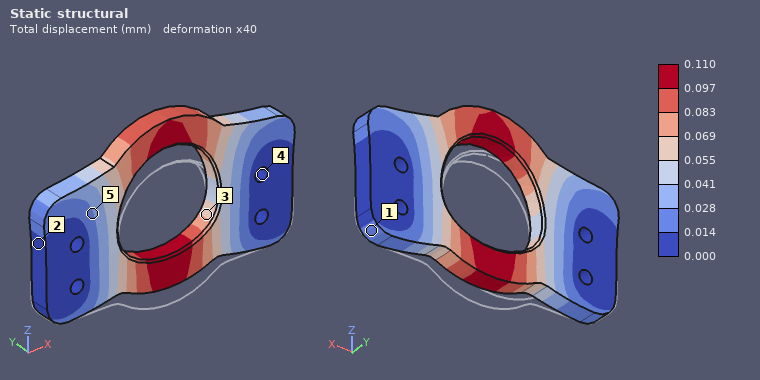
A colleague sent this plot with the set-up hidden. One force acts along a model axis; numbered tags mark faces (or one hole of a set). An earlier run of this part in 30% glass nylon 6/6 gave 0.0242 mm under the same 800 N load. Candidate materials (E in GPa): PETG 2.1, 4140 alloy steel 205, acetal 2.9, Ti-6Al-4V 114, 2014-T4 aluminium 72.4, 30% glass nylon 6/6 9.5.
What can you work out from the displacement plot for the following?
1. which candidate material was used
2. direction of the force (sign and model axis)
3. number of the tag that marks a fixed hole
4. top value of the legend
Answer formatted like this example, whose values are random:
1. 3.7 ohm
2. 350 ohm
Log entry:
1. PETG
2. +Z
3. 4
4. 0.110 mm
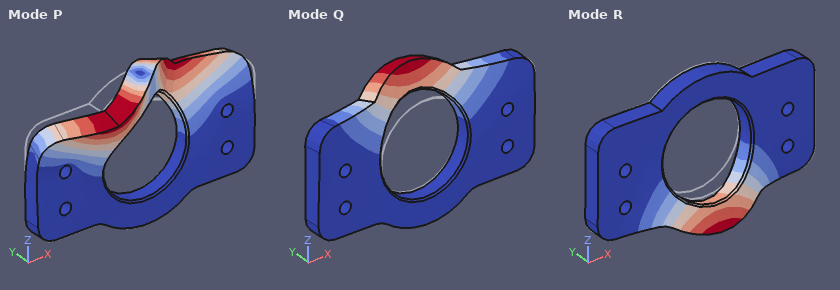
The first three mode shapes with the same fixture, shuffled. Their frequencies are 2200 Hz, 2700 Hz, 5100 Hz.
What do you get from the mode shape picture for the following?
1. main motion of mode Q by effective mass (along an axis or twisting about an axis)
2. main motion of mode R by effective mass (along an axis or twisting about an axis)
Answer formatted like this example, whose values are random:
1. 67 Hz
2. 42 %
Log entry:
1. along Y
2. along Y
